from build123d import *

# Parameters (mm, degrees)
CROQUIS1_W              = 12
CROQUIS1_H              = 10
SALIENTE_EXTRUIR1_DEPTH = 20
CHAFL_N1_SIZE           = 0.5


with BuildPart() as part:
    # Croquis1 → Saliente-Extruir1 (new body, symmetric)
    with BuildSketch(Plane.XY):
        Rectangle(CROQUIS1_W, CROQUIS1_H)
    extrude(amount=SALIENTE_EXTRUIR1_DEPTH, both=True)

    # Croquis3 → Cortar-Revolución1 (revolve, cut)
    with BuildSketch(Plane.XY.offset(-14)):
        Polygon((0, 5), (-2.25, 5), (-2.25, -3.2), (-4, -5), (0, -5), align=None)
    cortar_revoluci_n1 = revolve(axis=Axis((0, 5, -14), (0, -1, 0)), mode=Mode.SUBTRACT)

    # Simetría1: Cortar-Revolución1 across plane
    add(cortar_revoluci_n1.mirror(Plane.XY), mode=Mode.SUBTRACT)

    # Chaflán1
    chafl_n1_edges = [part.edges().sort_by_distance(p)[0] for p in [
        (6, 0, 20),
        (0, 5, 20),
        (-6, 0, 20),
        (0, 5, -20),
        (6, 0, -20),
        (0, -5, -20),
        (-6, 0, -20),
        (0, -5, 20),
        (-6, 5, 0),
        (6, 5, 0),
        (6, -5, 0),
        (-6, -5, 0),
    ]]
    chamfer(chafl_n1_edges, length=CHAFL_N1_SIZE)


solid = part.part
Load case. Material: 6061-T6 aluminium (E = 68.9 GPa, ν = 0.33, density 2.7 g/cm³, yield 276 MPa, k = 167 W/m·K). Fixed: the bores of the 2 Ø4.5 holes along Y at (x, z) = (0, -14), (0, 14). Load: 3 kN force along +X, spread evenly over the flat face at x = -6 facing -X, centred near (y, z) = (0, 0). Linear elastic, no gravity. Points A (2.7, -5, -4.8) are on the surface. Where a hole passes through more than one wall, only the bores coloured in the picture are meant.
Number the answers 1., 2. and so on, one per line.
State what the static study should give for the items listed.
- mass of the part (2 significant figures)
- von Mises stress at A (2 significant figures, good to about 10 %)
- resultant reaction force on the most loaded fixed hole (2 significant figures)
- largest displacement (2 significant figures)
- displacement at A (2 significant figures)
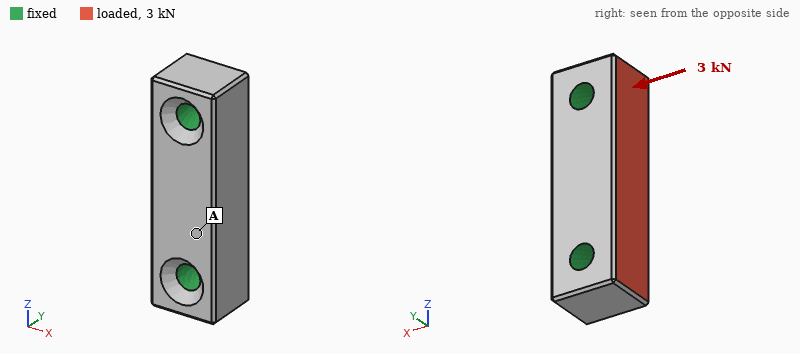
1. 12 g
2. 8.4 MPa
3. 1.5 kN
4. 4.8 µm
5. 3.8 µm
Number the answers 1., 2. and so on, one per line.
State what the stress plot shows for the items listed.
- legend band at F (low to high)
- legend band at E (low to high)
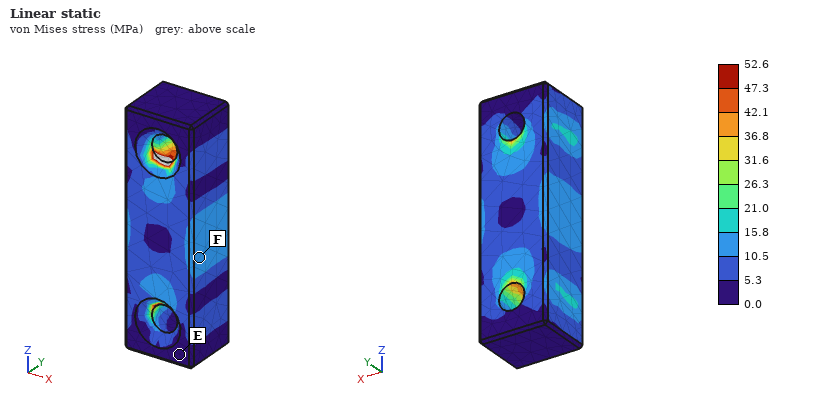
1. 10.5 to 15.8 MPa
2. 0.0 to 5.3 MPa
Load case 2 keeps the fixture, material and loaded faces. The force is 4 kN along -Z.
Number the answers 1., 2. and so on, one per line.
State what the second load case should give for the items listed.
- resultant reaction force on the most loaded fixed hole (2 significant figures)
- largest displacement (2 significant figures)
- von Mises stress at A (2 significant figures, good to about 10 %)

1. 2.1 kN
2. 4.6 µm
3. 5.1 MPa
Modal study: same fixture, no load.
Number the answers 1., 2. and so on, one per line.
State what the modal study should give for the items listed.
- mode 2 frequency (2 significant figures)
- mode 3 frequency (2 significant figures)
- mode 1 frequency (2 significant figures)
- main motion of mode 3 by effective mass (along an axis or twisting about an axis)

1. 41 kHz
2. 50 kHz
3. 40 kHz
4. twisting about Z
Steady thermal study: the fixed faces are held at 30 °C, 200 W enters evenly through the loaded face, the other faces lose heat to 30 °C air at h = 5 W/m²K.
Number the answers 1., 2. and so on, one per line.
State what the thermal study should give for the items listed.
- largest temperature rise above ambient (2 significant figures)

1. 38 K
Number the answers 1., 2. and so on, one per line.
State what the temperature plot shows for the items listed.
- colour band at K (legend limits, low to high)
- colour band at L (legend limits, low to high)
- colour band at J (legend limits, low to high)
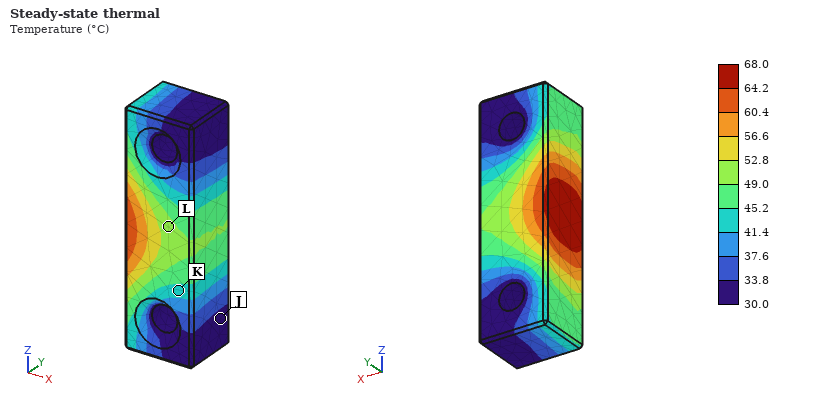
1. 41.4 to 45.2 °C
2. 49.0 to 52.8 °C
3. 30.0 to 33.8 °C
